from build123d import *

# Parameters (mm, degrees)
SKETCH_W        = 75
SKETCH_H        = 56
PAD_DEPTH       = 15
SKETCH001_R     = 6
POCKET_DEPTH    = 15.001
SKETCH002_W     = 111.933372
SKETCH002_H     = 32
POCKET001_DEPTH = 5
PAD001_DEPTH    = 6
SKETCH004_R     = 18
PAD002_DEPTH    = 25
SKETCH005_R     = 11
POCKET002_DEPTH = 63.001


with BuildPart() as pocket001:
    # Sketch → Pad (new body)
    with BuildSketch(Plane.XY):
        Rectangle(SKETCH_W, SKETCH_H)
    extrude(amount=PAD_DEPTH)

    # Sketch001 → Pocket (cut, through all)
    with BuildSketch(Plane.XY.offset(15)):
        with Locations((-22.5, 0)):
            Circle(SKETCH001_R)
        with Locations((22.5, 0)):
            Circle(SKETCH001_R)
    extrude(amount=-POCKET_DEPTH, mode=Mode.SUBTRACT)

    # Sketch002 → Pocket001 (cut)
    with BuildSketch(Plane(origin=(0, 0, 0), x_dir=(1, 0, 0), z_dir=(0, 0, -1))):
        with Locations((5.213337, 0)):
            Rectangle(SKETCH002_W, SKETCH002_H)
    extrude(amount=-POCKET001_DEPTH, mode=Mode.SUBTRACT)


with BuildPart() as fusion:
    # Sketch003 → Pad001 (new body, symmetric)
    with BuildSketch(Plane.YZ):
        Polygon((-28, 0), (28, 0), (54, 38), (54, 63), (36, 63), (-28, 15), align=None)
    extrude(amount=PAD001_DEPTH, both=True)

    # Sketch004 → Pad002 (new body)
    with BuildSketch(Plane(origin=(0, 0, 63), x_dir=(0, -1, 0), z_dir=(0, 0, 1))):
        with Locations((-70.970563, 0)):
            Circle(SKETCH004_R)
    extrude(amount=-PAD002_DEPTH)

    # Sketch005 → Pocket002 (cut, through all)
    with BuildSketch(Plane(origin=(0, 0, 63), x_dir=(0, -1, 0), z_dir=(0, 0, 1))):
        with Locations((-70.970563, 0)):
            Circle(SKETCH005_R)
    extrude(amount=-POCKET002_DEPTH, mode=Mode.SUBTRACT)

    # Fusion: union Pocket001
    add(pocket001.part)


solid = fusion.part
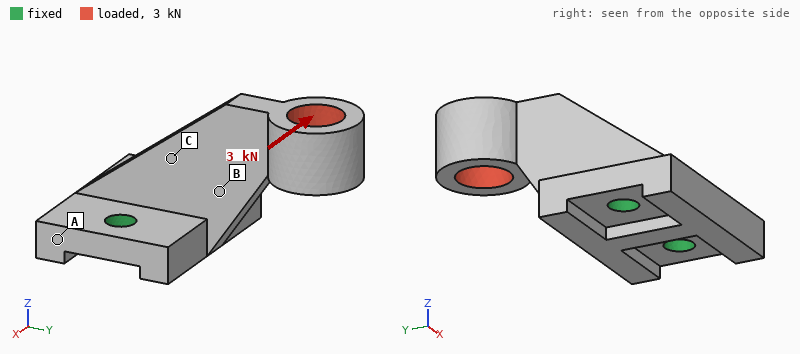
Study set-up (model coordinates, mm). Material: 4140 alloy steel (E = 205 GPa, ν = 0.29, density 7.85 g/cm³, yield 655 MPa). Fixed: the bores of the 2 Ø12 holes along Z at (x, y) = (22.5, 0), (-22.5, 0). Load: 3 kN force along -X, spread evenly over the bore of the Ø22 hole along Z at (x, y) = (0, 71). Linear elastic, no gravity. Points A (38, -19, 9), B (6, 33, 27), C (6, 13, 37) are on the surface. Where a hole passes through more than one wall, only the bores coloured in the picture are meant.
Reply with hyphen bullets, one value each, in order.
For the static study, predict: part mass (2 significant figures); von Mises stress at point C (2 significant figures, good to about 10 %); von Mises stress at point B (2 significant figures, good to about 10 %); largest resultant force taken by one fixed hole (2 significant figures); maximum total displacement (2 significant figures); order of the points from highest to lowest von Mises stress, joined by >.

- 740 g
- 130 MPa
- 160 MPa
- 5.4 kN
- 0.46 mm
- B > C > A
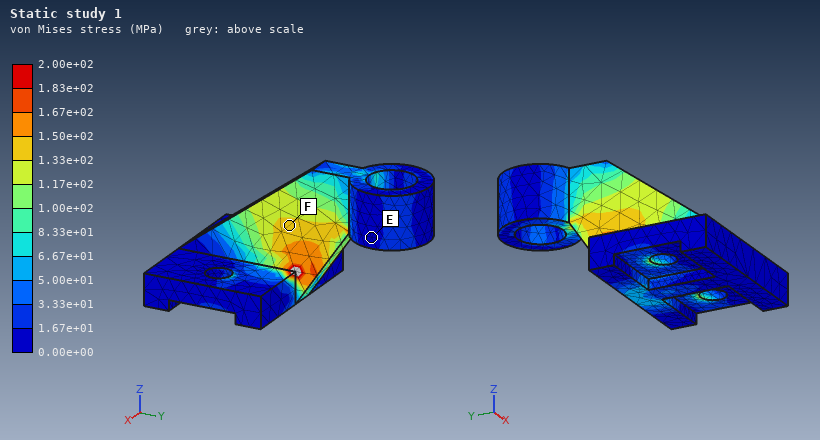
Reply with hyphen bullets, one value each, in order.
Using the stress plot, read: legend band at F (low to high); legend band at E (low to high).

- 1.33e+02 to 1.50e+02 MPa
- 0.00e+00 to 1.67e+01 MPa
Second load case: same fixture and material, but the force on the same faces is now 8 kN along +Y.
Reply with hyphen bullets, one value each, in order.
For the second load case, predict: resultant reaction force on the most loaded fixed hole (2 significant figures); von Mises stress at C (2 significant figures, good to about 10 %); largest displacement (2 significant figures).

- 4.0 kN
- 52 MPa
- 0.20 mm
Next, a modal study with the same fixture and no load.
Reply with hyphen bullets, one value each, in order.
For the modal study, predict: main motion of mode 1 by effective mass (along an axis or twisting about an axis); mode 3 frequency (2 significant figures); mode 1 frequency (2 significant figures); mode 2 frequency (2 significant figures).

- along X
- 3700 Hz
- 1300 Hz
- 1900 Hz
